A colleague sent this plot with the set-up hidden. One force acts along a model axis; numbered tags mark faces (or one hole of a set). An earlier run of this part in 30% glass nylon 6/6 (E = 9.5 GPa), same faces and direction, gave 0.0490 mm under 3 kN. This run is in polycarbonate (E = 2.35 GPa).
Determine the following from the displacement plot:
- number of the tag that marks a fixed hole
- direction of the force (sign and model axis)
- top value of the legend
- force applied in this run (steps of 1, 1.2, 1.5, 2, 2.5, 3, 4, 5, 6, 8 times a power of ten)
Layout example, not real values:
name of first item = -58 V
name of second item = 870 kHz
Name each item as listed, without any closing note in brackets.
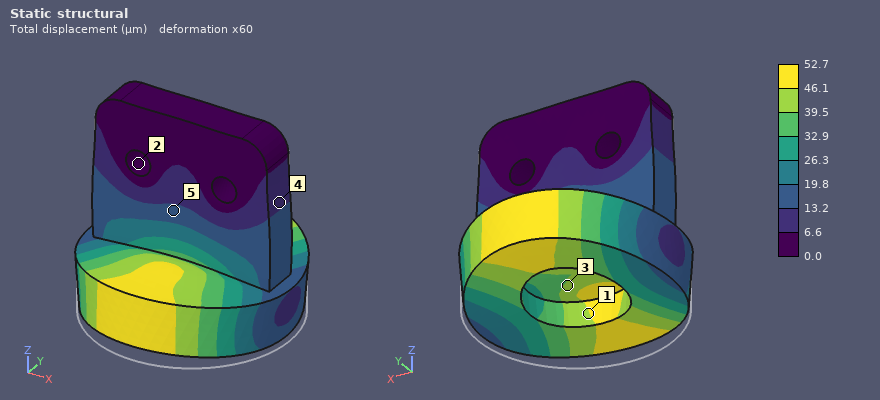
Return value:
number of the tag that marks a fixed hole = 2
direction of the force = +Z
top value of the legend = 52.7 µm
force applied in this run = 800 N
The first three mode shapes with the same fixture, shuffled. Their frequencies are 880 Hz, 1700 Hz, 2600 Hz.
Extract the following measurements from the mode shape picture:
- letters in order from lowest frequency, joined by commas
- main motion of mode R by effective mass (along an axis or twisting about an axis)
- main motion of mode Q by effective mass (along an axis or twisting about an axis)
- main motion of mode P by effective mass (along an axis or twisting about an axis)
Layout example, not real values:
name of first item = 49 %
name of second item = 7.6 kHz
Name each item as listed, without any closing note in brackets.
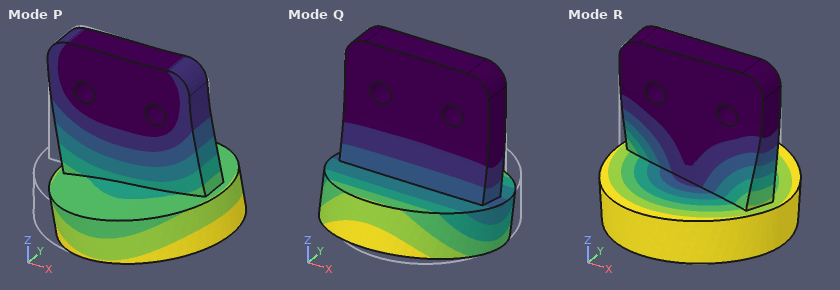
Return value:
letters in order from lowest frequency, joined by commas = Q, R, P
main motion of mode R by effective mass = twisting about Z
main motion of mode Q by effective mass = along Y
main motion of mode P by effective mass = along X
